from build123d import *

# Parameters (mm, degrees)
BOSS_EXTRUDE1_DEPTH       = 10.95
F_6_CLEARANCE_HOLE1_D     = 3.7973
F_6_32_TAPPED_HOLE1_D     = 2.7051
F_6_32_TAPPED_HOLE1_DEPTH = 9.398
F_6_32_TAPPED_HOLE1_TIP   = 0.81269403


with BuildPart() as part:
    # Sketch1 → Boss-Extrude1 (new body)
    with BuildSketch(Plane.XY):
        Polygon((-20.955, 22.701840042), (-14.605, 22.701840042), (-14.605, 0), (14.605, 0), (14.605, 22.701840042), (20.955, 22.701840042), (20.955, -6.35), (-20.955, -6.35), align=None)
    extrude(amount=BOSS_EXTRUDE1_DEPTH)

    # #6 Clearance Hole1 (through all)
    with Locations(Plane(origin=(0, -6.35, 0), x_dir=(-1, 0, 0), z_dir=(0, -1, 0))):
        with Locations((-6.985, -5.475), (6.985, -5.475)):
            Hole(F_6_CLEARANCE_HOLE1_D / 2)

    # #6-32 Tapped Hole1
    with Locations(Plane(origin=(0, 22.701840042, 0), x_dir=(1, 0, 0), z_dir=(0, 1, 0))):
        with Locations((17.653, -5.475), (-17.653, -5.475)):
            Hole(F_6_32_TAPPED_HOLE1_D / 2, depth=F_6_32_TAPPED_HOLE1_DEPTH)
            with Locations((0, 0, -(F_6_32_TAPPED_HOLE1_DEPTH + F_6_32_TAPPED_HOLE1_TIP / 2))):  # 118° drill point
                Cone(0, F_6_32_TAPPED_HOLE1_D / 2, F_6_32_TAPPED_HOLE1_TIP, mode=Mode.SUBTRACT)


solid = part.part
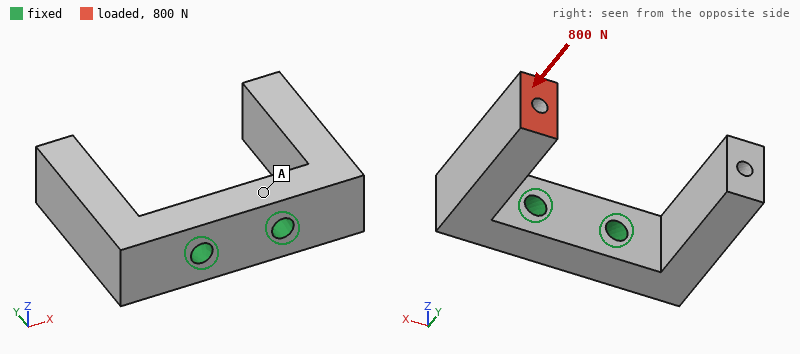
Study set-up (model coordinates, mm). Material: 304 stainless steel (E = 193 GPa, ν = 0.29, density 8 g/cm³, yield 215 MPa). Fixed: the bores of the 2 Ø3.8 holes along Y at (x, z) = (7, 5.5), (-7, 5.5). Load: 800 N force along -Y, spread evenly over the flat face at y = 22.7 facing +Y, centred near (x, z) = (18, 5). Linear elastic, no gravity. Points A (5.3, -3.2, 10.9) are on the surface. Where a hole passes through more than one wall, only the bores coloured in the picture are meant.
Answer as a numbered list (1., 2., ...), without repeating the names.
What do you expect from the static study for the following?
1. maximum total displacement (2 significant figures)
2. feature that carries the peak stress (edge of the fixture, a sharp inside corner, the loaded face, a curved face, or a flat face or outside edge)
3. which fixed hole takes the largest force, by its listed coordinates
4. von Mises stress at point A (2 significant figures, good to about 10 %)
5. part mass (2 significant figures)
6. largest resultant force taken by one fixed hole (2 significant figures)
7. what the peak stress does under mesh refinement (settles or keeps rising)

1. 29 µm
2. edge of the fixture
3. (7, 5.5)
4. 15 MPa
5. 47 g
6. 880 N
7. keeps rising
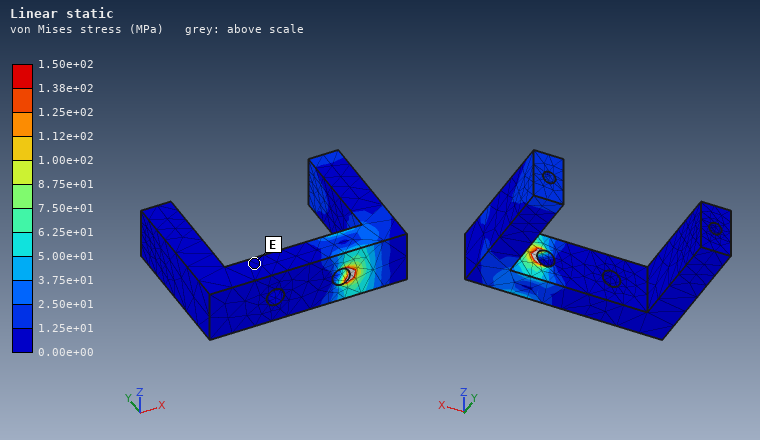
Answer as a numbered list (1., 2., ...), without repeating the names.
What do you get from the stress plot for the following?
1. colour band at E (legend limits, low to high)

1. 0.00e+00 to 1.25e+01 MPa
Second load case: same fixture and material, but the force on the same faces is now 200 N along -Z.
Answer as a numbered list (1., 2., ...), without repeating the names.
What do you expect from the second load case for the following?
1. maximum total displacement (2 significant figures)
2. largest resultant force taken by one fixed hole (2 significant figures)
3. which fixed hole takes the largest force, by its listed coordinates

1. 34 µm
2. 260 N
3. (7, 5.5)
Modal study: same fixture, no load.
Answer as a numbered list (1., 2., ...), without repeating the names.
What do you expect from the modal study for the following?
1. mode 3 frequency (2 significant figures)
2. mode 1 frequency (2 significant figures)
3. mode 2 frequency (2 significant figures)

1. 5800 Hz
2. 4900 Hz
3. 4900 Hz
